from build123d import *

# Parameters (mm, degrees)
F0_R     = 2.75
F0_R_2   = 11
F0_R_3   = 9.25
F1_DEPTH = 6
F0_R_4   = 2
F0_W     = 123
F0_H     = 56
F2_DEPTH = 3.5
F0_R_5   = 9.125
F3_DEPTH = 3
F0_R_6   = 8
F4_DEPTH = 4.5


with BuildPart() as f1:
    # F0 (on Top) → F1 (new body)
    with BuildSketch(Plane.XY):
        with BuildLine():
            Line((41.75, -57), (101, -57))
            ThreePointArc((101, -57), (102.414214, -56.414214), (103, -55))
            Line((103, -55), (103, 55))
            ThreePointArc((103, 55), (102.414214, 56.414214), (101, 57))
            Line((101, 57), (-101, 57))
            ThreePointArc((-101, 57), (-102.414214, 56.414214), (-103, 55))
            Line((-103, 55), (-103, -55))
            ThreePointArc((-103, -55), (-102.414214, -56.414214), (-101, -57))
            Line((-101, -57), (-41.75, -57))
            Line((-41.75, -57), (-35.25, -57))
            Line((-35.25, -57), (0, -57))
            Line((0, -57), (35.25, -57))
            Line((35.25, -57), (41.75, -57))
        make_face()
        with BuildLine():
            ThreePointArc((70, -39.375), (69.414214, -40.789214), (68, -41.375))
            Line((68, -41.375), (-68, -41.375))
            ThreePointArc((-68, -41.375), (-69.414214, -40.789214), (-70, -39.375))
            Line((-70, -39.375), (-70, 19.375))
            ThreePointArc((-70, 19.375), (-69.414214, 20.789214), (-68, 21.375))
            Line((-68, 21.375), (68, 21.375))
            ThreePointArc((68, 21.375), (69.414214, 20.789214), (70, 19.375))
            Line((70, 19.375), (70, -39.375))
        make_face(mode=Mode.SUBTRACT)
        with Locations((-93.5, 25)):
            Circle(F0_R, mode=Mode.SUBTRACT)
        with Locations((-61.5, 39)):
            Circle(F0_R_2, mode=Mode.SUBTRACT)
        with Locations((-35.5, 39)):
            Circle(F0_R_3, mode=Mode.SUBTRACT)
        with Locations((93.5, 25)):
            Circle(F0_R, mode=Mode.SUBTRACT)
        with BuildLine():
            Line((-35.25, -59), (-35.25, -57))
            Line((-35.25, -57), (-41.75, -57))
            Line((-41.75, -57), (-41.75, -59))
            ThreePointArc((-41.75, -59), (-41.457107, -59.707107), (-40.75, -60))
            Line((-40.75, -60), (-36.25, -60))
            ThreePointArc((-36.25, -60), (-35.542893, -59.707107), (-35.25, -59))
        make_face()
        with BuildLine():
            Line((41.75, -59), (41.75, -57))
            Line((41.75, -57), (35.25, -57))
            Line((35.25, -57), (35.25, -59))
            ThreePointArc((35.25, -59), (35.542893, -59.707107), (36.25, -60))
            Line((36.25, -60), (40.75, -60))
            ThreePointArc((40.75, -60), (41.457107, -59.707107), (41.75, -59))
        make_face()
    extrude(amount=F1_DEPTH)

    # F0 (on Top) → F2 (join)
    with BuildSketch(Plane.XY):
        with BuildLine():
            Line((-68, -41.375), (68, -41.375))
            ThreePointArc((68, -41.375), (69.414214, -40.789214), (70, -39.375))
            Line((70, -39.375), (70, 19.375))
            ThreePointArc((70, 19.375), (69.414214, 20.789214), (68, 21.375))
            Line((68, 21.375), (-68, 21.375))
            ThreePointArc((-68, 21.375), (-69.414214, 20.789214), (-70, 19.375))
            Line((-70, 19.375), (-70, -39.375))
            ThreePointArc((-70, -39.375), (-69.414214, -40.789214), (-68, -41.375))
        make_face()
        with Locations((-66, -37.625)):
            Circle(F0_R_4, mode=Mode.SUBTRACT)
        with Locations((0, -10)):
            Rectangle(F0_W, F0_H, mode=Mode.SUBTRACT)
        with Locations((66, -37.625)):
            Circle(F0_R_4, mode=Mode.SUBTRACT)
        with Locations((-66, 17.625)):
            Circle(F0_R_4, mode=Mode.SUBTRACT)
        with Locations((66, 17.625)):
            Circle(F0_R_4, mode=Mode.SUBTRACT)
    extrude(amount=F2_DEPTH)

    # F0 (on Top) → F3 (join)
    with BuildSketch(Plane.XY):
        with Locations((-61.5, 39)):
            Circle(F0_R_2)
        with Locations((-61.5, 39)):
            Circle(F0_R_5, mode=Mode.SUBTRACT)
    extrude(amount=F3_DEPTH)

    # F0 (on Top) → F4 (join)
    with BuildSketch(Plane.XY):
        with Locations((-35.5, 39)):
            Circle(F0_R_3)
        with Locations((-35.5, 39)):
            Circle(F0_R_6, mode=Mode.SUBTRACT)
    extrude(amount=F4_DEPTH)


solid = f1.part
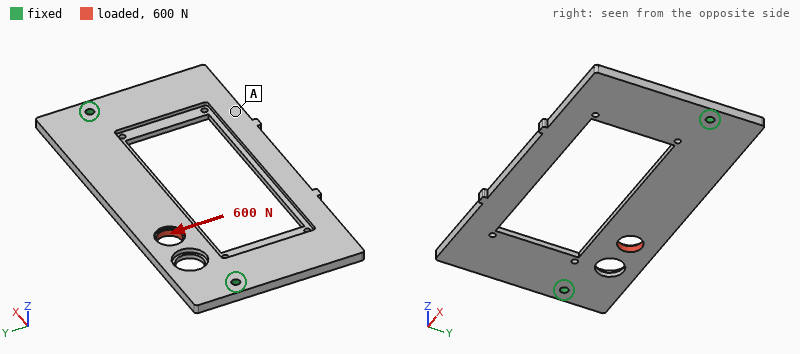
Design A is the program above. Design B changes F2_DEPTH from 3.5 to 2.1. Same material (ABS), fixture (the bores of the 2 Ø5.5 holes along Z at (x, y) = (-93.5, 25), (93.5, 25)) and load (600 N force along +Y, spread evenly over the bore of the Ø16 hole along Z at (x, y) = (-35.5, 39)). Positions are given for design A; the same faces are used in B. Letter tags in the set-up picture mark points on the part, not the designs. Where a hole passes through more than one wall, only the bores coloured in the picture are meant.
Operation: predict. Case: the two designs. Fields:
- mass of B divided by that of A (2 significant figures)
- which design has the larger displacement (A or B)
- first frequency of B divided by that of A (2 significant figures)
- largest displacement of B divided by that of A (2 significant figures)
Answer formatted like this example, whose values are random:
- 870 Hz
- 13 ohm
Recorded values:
- 0.97
- B
- 1.0
- 1.1
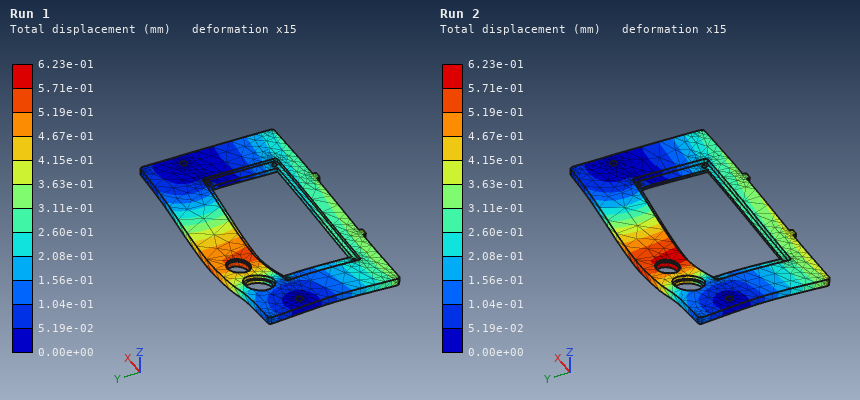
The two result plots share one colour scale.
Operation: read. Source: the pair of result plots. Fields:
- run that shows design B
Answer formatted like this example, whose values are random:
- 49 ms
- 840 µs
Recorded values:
- Run 2
